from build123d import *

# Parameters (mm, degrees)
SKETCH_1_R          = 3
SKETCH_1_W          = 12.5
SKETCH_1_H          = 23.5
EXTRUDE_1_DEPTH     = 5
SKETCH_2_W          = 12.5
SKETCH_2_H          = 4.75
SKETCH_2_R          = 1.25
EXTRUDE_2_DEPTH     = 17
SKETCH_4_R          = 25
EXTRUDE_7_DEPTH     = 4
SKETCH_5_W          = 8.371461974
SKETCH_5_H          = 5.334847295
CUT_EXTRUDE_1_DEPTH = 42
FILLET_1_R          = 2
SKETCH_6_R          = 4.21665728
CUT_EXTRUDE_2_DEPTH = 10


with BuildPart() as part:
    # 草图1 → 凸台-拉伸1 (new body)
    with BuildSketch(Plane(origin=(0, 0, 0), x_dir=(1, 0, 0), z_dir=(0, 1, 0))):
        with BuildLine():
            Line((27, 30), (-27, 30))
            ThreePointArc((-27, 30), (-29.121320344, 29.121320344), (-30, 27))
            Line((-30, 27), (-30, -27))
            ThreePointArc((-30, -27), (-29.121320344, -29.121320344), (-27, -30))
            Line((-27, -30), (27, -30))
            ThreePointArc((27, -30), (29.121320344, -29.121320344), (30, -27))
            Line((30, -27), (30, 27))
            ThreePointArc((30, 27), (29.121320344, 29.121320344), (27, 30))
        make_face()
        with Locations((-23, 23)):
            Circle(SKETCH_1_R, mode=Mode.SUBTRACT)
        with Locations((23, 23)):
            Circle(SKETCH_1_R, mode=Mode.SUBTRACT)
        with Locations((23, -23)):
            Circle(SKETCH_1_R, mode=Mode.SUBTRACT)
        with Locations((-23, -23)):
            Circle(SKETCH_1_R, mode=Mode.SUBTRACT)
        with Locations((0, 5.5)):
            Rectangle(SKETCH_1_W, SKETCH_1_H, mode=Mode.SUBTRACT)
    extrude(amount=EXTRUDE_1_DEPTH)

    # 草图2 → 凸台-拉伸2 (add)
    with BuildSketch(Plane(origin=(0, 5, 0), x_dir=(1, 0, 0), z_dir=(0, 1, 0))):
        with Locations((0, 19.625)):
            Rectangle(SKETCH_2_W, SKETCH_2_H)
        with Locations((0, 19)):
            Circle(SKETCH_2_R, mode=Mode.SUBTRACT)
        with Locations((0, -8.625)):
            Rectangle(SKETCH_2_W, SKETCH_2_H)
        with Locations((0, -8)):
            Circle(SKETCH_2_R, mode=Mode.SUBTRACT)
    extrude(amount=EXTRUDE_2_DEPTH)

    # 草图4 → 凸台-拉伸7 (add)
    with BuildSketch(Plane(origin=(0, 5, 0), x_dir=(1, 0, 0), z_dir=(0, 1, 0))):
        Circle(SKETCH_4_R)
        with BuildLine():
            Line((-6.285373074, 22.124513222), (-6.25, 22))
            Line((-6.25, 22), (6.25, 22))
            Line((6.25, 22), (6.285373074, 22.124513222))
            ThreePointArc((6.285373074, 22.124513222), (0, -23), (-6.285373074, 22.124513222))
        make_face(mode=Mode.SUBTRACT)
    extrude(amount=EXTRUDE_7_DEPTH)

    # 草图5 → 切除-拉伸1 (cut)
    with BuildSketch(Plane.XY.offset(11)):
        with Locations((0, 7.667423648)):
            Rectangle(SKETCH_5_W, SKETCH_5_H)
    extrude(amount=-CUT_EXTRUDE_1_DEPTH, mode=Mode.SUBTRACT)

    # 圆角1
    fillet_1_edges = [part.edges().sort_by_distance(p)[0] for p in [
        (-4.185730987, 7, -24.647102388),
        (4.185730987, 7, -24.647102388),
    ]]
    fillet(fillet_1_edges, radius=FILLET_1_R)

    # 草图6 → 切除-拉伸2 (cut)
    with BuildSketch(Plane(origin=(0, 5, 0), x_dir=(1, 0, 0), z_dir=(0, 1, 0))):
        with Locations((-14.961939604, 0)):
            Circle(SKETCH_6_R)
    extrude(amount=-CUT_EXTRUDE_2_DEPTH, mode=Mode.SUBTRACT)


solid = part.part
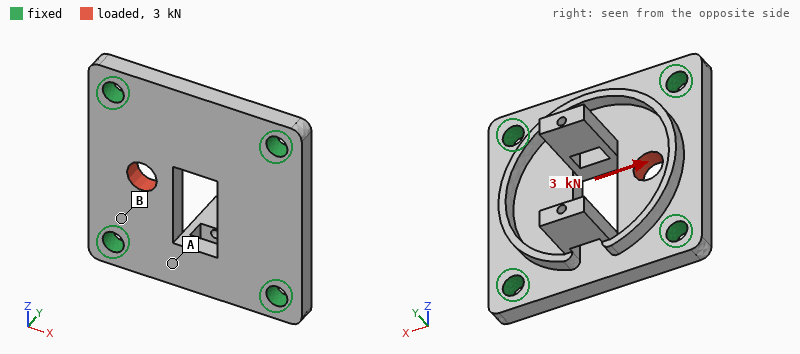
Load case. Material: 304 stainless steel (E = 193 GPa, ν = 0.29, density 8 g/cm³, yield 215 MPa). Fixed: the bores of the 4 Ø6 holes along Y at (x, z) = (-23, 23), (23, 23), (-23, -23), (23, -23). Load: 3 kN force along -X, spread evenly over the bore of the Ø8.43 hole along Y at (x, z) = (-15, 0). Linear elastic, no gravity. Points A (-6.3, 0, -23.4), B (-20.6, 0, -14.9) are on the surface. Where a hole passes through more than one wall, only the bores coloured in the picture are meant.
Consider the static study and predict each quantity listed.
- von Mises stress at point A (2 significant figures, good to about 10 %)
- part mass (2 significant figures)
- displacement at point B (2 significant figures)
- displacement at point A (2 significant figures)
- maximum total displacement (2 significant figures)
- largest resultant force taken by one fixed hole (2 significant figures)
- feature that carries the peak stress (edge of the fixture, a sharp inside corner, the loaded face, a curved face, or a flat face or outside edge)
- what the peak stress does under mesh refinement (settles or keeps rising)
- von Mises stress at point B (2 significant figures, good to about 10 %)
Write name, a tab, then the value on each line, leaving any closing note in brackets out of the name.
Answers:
von Mises stress at point A	5.8 MPa
part mass	150 g
displacement at point B	1.8 µm
displacement at point A	1.4 µm
maximum total displacement	5.5 µm
largest resultant force taken by one fixed hole	1.2 kN
feature that carries the peak stress	a sharp inside corner
what the peak stress does under mesh refinement	keeps rising
von Mises stress at point B	25 MPa
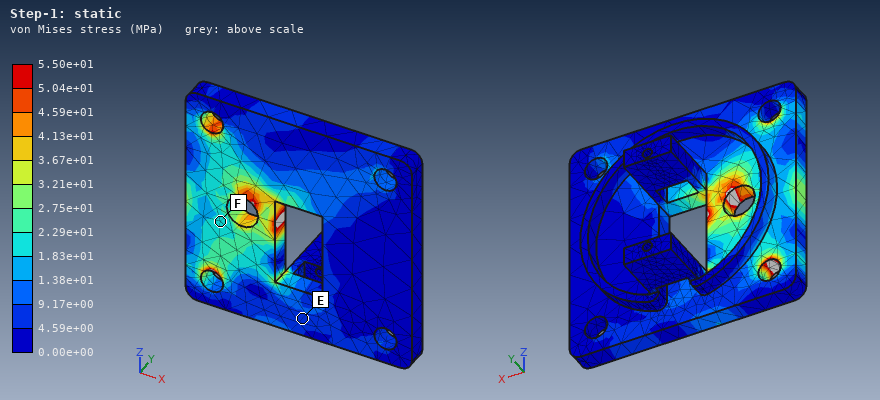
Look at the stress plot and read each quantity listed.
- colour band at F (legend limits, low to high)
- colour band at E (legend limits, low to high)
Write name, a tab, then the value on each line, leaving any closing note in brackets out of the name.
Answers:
colour band at F	1.83e+01 to 2.29e+01 MPa
colour band at E	4.59e+00 to 9.17e+00 MPa
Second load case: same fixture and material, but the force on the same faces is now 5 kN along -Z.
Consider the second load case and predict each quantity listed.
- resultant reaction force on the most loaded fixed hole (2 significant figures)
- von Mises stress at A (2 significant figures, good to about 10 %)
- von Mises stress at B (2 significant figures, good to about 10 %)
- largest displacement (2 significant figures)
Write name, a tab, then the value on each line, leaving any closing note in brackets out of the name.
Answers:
resultant reaction force on the most loaded fixed hole	2.3 kN
von Mises stress at A	6.7 MPa
von Mises stress at B	32 MPa
largest displacement	4.3 µm
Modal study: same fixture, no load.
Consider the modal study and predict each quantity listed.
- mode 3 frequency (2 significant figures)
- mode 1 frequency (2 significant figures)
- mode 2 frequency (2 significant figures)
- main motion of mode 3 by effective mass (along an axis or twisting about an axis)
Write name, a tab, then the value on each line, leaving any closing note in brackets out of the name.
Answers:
mode 3 frequency	9200 Hz
mode 1 frequency	6200 Hz
mode 2 frequency	7400 Hz
main motion of mode 3 by effective mass	along Y
